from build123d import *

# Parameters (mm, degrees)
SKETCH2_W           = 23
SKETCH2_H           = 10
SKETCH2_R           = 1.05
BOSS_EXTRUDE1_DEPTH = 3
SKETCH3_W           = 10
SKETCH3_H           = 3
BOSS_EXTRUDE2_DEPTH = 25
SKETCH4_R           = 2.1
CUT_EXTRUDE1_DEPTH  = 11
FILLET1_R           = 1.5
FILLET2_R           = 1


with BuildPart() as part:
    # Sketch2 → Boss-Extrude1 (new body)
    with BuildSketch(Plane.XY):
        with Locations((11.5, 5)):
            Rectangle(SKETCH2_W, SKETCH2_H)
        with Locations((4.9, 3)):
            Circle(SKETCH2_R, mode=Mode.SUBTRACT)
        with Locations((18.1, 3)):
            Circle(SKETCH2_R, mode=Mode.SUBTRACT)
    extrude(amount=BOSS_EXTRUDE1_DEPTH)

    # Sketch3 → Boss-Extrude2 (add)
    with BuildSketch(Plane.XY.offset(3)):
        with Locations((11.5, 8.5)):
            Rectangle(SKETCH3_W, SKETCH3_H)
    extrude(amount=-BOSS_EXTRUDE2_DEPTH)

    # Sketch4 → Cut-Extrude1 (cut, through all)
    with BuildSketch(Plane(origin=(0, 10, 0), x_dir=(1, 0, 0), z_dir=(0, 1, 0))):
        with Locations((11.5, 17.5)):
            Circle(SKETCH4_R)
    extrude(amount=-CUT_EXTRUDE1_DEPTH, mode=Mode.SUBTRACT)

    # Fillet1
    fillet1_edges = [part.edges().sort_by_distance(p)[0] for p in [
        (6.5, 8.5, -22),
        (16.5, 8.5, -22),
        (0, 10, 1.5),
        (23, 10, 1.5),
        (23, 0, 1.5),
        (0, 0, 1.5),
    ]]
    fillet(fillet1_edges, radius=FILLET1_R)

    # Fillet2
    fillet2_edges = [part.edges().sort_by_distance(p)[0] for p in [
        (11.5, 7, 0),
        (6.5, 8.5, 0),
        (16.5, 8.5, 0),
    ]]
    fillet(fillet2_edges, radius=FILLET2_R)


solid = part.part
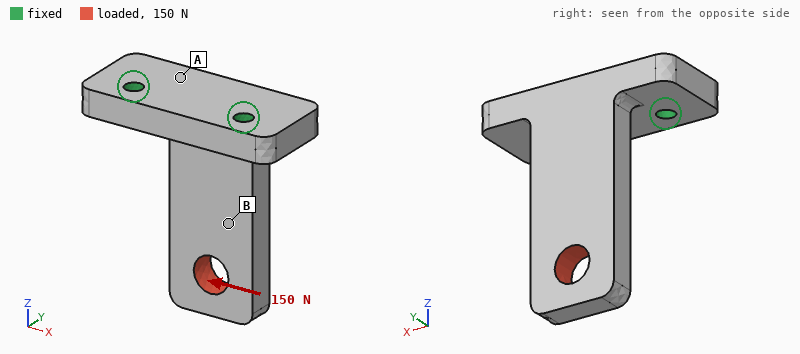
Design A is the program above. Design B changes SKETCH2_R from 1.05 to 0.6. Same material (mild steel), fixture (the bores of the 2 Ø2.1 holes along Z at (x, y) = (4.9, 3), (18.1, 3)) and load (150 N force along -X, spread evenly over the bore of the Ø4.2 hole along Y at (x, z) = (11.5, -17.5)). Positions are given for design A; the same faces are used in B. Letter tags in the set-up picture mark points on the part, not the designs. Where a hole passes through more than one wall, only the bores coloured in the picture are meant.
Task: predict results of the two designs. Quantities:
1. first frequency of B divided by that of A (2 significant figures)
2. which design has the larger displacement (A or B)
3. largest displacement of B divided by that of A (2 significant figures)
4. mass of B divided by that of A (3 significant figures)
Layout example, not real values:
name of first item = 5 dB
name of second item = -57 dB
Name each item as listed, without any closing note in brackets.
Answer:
first frequency of B divided by that of A = 0.96
which design has the larger displacement = B
largest displacement of B divided by that of A = 1.1
mass of B divided by that of A = 1.01
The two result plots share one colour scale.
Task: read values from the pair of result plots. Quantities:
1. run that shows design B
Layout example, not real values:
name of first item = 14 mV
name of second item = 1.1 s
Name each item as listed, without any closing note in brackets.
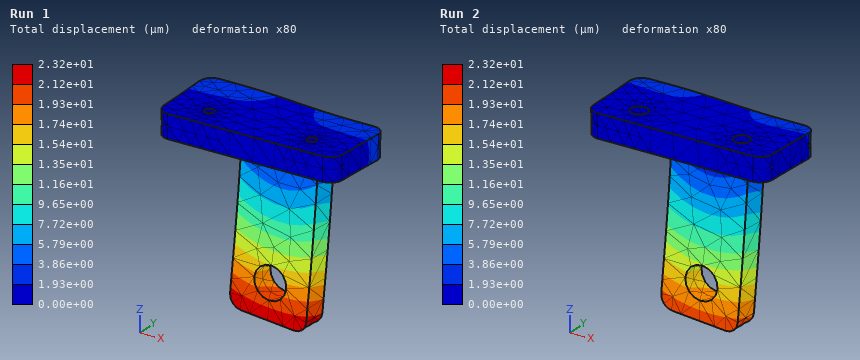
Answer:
run that shows design B = Run 1
